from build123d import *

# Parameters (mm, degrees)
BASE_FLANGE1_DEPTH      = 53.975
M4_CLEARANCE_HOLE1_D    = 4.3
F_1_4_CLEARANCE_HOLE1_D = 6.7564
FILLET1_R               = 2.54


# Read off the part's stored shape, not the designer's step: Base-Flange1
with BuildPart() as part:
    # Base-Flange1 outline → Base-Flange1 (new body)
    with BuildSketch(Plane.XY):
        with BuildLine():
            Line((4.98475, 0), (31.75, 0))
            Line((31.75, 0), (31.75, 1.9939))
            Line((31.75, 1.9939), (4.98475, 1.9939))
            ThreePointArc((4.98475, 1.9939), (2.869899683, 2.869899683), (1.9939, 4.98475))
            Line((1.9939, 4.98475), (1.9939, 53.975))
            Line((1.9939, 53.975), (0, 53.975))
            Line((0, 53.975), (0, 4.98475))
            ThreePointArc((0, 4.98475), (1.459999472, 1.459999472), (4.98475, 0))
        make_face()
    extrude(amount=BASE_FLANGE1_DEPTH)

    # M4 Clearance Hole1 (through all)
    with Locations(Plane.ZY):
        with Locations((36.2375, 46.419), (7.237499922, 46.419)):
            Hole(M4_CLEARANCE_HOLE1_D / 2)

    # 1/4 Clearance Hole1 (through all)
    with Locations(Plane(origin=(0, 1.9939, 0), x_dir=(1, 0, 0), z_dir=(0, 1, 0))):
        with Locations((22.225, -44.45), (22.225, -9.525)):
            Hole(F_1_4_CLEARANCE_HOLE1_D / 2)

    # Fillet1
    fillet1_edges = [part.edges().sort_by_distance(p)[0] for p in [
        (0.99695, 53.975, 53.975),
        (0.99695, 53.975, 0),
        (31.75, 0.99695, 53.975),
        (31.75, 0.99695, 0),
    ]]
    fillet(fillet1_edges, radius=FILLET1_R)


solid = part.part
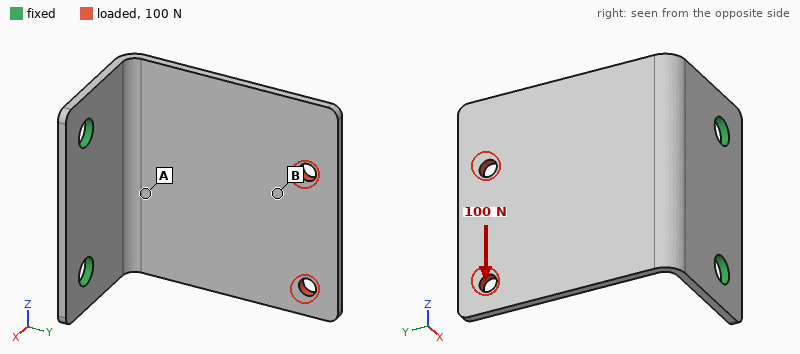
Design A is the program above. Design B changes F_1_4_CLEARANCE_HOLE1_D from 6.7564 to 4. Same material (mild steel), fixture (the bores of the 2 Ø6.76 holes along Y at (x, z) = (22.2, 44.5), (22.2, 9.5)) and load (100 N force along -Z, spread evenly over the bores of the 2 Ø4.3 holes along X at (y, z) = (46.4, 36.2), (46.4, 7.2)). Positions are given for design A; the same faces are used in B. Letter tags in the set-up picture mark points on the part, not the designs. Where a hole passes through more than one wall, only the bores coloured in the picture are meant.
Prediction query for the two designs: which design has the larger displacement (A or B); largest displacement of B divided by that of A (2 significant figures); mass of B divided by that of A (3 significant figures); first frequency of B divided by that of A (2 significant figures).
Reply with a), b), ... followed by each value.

a) B
b) 1.2
c) 1.01
d) 0.96
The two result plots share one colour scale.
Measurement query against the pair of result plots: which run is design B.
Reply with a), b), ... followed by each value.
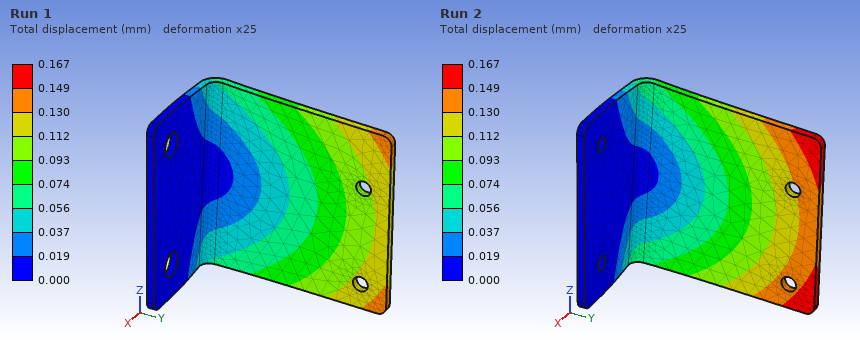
a) Run 2
